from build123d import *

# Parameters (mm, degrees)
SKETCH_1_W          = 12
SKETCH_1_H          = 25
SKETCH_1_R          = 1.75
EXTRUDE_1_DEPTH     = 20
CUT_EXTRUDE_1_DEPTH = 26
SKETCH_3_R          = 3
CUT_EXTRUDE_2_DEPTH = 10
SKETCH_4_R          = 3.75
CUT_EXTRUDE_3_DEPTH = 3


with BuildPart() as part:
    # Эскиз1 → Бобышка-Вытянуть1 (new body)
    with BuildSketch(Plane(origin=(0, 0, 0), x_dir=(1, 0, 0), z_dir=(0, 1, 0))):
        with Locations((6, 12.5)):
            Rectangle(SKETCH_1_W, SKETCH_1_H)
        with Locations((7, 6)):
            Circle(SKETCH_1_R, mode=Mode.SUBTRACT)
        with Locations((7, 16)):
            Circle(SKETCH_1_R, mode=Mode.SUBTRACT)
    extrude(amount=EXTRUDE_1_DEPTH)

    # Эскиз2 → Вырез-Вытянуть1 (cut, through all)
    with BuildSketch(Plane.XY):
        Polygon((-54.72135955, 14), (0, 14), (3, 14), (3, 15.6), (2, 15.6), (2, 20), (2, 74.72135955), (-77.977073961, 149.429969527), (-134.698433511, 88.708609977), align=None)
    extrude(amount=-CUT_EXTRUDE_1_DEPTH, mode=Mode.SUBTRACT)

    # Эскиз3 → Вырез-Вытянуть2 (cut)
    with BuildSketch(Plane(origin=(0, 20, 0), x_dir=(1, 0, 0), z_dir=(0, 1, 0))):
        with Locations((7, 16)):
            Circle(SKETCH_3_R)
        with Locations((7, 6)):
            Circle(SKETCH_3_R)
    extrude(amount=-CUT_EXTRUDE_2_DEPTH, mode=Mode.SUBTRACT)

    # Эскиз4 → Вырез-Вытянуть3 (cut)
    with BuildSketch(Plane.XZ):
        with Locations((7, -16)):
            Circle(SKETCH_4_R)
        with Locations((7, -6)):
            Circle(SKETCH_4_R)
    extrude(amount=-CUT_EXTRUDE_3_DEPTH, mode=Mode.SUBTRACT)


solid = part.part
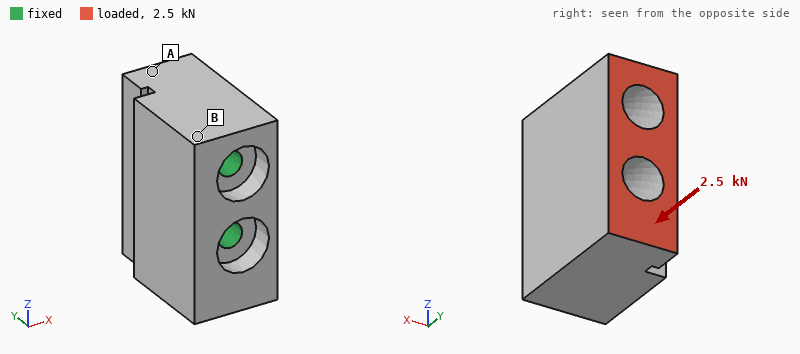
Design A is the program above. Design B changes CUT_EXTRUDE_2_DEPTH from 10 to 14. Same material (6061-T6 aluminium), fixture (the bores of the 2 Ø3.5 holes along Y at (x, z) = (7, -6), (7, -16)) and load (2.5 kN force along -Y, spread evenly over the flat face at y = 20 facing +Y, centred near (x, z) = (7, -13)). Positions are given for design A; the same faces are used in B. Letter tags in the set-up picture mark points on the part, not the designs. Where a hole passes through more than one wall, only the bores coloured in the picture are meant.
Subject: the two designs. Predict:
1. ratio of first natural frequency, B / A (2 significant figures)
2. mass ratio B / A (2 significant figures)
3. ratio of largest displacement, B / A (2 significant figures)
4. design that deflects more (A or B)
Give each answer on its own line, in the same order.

0.44
0.97
1.7
B
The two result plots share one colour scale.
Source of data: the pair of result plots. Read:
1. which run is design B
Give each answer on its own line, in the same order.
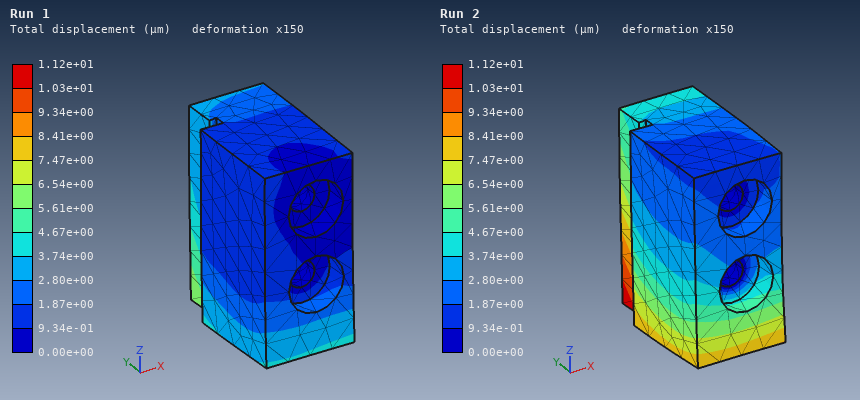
Run 2
